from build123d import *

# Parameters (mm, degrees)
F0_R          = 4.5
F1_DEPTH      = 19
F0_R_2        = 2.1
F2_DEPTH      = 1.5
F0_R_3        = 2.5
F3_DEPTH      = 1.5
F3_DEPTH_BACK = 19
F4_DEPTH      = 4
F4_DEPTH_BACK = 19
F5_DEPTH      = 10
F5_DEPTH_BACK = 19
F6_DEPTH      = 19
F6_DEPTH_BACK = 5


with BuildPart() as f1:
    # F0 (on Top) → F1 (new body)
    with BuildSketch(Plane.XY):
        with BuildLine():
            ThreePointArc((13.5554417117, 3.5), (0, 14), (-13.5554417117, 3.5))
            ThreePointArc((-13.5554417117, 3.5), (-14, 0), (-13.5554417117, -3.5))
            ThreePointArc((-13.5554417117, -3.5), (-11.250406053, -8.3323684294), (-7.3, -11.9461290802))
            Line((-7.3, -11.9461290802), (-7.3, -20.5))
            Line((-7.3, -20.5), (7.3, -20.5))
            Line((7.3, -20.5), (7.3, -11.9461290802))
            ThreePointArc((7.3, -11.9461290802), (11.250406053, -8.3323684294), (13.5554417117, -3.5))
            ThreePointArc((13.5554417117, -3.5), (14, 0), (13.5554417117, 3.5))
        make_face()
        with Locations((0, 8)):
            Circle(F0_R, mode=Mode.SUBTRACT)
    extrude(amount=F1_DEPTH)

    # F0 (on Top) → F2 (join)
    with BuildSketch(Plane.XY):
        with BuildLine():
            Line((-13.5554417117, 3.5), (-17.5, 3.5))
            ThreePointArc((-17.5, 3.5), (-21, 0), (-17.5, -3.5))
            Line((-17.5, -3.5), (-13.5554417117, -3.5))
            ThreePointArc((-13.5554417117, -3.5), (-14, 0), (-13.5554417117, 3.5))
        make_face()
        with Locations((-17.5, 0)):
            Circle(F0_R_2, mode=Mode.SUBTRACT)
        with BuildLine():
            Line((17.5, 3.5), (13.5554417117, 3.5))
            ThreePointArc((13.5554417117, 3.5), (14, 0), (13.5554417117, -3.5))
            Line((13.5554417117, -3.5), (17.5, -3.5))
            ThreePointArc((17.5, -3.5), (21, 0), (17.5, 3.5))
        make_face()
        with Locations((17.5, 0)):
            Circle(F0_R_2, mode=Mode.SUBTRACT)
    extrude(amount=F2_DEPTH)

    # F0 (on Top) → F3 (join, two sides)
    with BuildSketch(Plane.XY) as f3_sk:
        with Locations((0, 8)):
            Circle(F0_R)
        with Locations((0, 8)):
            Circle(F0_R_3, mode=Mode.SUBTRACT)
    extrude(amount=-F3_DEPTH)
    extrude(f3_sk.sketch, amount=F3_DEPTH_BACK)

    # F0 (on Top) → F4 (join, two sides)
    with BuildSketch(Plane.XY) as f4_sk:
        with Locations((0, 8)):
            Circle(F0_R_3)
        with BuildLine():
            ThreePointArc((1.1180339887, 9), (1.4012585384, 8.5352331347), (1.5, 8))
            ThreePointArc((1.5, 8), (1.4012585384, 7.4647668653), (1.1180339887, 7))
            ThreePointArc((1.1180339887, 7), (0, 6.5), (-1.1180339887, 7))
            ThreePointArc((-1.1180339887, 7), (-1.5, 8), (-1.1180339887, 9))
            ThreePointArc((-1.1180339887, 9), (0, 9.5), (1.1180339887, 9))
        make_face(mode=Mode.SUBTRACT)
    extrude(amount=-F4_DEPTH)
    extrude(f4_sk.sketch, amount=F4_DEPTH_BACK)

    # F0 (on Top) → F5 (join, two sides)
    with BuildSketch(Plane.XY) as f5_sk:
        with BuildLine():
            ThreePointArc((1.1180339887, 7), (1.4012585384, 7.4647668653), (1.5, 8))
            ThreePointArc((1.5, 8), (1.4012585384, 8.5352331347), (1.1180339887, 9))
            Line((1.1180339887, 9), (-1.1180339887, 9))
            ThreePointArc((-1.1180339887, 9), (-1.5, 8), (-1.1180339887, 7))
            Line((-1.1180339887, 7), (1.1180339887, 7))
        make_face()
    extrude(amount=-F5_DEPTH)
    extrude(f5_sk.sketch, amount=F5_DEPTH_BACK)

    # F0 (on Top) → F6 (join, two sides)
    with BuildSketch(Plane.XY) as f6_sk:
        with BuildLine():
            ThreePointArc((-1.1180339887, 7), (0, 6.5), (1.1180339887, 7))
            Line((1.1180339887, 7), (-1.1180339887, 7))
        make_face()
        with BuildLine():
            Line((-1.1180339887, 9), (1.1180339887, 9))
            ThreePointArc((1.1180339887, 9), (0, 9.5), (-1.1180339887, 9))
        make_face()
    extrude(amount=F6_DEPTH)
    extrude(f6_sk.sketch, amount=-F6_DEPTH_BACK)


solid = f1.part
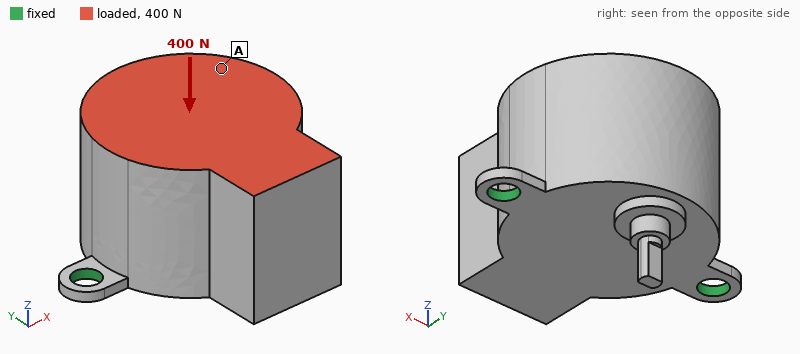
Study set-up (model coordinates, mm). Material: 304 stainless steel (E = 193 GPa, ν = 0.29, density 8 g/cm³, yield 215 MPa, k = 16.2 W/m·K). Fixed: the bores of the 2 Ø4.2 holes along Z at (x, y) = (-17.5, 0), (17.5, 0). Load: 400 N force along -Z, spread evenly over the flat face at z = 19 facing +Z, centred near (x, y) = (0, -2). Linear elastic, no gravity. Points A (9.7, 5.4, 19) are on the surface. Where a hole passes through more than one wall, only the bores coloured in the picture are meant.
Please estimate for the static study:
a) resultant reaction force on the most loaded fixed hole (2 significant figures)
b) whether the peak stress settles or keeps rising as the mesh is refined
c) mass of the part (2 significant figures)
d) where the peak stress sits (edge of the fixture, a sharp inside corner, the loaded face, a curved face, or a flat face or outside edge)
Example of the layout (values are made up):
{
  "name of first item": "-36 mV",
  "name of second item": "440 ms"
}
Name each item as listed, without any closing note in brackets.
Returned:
{
  "resultant reaction force on the most loaded fixed hole": "230 N",
  "whether the peak stress settles or keeps rising as the mesh is refined": "keeps rising",
  "mass of the part": "110 g",
  "where the peak stress sits": "edge of the fixture"
}
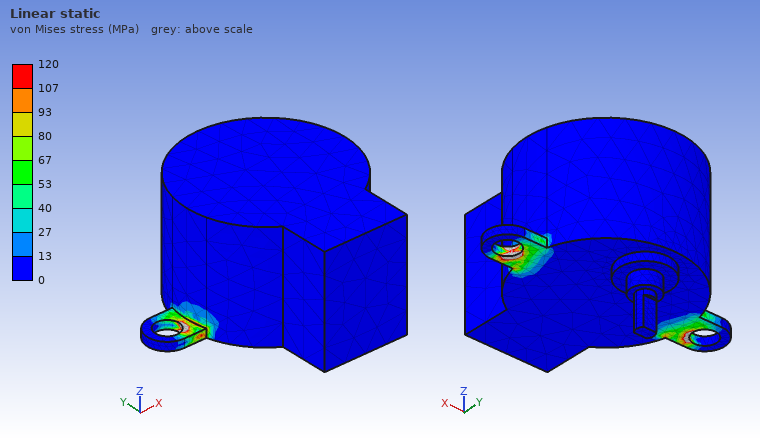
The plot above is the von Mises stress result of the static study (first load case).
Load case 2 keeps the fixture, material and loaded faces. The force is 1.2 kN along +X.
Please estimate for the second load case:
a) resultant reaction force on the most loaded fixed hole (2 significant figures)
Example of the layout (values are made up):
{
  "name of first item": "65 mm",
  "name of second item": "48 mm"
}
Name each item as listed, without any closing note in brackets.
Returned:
{
  "resultant reaction force on the most loaded fixed hole": "960 N"
}
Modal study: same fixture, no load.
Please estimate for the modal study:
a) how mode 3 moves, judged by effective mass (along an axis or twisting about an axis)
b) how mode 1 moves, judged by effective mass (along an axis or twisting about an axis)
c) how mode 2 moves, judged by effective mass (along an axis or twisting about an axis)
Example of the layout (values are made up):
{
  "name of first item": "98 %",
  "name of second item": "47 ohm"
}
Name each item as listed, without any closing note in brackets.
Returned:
{
  "how mode 3 moves, judged by effective mass": "along X",
  "how mode 1 moves, judged by effective mass": "along Y",
  "how mode 2 moves, judged by effective mass": "along Z"
}
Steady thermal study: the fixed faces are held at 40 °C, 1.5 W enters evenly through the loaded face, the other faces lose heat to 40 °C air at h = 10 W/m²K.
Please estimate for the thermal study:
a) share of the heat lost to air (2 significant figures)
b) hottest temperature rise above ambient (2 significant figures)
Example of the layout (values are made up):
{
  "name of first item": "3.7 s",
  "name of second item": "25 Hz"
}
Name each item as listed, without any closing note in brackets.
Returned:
{
  "share of the heat lost to air": "25 %",
  "hottest temperature rise above ambient": "15 K"
}
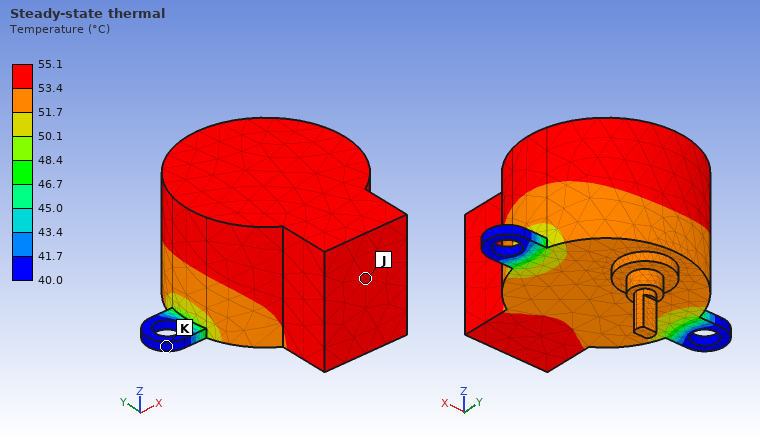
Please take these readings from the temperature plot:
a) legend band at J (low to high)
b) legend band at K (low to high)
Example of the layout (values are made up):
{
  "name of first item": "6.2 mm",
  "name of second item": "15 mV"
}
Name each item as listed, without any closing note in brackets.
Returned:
{
  "legend band at J": "53.4 to 55.1 °C",
  "legend band at K": "40.0 to 41.7 °C"
}
